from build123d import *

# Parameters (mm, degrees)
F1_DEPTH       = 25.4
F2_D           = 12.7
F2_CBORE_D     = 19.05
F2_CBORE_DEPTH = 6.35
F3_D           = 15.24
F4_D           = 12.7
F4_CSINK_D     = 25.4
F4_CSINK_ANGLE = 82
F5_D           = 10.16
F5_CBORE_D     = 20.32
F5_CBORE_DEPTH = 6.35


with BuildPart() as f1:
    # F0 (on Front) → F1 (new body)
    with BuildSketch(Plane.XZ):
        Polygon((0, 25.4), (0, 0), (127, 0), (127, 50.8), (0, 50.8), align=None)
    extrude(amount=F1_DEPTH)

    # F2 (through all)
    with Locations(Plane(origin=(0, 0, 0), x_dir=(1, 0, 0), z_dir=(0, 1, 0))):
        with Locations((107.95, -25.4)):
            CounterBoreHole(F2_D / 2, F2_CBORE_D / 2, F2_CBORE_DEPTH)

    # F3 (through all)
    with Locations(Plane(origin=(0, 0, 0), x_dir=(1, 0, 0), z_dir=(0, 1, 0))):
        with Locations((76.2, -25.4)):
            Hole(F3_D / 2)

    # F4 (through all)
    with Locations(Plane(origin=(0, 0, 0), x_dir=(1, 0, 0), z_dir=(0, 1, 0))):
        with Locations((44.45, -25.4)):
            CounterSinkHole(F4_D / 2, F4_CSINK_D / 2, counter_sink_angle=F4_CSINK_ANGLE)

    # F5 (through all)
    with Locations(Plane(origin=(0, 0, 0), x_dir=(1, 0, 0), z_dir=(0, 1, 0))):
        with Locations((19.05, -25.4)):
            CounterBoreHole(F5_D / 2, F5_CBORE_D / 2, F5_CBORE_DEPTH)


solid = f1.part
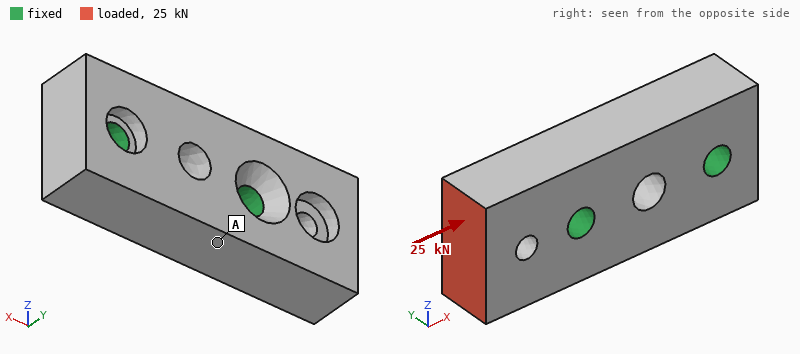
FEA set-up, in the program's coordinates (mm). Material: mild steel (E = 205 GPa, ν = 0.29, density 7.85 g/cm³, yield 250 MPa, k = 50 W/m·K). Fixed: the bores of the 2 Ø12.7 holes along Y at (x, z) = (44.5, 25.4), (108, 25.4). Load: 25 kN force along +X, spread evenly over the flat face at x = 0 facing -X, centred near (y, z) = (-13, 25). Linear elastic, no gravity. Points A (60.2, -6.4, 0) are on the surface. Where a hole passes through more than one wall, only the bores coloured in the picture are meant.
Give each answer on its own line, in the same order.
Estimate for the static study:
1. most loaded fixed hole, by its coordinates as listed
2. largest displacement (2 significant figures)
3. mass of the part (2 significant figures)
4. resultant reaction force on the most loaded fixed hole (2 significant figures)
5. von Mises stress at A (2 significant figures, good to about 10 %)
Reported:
(44.5, 25.4)
11 µm
1.2 kg
21 kN
12 MPa
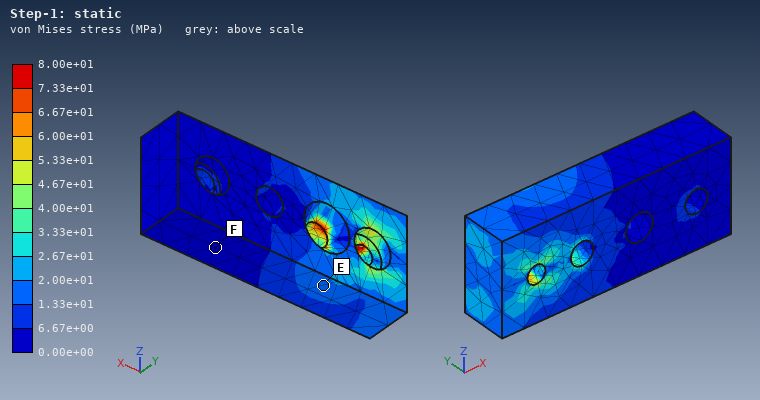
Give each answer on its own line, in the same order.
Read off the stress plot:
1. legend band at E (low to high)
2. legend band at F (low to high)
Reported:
1.33e+01 to 2.00e+01 MPa
0.00e+00 to 6.67e+00 MPa
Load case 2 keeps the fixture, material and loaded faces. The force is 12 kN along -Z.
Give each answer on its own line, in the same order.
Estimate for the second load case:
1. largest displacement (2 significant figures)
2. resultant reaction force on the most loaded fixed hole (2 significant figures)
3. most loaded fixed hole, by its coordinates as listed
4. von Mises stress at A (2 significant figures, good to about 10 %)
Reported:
29 µm
17 kN
(44.5, 25.4)
30 MPa
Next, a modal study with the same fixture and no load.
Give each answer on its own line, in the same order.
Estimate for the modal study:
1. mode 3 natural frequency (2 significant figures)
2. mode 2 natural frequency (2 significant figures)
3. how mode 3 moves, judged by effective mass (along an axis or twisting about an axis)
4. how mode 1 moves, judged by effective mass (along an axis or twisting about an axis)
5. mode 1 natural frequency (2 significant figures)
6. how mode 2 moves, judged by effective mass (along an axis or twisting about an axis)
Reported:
10 kHz
8800 Hz
twisting about X
along Y
7200 Hz
along Z
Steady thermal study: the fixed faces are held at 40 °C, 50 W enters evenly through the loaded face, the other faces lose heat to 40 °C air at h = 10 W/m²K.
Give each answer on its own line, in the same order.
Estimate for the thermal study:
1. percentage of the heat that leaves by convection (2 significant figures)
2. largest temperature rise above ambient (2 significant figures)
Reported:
3.7 %
42 K
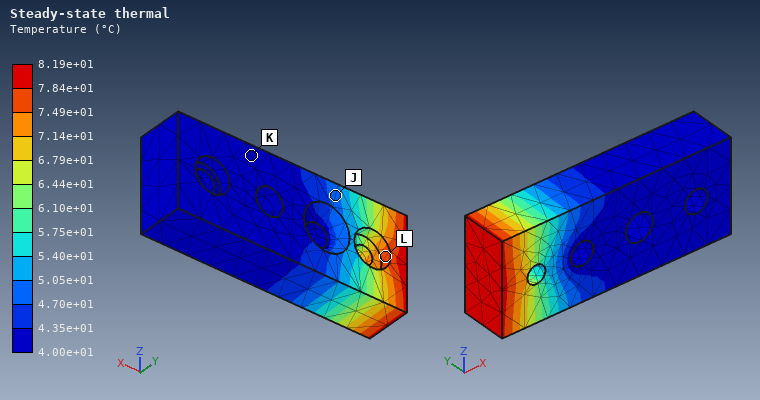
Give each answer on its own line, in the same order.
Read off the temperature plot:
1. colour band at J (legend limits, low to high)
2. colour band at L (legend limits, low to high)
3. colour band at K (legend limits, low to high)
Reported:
4.70e+01 to 5.05e+01 °C
7.49e+01 to 7.84e+01 °C
4.00e+01 to 4.35e+01 °C
